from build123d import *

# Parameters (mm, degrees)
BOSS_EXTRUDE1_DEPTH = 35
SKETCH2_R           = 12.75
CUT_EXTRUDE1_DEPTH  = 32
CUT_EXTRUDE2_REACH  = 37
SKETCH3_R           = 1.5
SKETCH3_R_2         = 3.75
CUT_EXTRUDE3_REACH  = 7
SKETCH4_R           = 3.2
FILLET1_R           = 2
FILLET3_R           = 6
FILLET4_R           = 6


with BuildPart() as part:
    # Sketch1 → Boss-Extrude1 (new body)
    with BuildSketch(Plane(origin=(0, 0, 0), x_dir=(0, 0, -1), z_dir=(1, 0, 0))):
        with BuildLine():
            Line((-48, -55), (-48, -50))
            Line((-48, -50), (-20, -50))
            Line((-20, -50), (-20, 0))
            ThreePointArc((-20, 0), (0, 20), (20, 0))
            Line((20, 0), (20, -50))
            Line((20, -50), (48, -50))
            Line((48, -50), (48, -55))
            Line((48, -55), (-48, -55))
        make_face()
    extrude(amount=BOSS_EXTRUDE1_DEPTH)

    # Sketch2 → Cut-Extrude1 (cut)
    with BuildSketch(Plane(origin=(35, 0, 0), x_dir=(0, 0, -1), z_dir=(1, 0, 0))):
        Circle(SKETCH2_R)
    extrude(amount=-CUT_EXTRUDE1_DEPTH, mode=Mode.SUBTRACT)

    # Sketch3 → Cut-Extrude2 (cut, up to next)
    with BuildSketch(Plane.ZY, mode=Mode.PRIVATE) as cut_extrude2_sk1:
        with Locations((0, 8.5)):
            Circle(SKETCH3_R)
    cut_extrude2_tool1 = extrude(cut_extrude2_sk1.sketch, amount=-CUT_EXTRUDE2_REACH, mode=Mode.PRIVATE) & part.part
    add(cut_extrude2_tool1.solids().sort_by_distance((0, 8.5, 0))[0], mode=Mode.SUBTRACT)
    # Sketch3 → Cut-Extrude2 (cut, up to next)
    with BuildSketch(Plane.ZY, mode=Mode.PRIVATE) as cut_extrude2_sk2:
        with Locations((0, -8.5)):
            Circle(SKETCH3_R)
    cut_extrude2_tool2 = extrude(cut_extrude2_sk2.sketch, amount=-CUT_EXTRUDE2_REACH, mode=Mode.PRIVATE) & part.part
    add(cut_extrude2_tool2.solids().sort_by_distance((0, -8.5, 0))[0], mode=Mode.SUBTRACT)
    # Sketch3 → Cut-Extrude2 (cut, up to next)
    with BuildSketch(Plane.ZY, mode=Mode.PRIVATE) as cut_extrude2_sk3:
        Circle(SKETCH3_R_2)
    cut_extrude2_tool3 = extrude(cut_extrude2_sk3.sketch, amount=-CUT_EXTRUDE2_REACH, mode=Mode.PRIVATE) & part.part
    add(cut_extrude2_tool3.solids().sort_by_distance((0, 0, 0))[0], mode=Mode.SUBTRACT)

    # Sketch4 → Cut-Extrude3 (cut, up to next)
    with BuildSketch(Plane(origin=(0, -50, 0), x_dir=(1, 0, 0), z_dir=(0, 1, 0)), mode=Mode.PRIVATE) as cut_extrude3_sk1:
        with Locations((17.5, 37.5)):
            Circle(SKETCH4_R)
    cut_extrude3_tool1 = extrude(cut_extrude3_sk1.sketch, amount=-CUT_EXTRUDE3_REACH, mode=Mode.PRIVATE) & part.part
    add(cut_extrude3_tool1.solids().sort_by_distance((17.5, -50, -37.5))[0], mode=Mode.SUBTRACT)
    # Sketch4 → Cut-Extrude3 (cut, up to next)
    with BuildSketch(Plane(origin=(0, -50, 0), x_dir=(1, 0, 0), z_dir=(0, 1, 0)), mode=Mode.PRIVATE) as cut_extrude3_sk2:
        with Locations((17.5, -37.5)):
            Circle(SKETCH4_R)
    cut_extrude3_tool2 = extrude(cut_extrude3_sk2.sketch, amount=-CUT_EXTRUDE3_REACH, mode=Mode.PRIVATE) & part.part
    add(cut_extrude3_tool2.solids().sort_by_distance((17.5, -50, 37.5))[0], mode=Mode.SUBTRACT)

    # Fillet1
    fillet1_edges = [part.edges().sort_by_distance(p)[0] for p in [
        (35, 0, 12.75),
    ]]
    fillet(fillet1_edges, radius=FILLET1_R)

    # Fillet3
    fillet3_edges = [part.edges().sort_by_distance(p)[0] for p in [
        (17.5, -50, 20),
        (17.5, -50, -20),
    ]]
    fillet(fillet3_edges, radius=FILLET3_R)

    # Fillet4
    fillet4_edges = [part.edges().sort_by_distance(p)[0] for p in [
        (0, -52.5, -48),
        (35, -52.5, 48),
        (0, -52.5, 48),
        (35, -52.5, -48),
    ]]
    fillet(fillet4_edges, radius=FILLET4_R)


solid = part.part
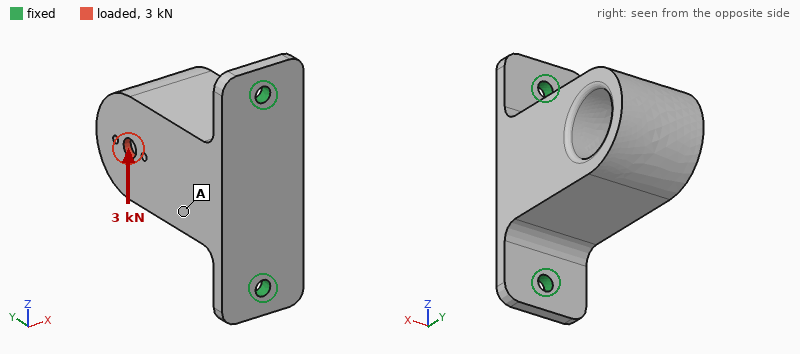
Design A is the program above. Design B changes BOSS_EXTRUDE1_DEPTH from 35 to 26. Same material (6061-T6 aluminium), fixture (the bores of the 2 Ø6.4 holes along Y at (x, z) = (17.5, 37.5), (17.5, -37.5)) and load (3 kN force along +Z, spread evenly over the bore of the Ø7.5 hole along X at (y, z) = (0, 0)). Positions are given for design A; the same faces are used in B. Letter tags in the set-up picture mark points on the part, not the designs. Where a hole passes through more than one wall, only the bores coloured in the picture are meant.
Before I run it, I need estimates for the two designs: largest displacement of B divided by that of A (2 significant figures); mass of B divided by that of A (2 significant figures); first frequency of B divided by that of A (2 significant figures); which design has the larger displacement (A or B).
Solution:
1.2
0.75
0.97
B
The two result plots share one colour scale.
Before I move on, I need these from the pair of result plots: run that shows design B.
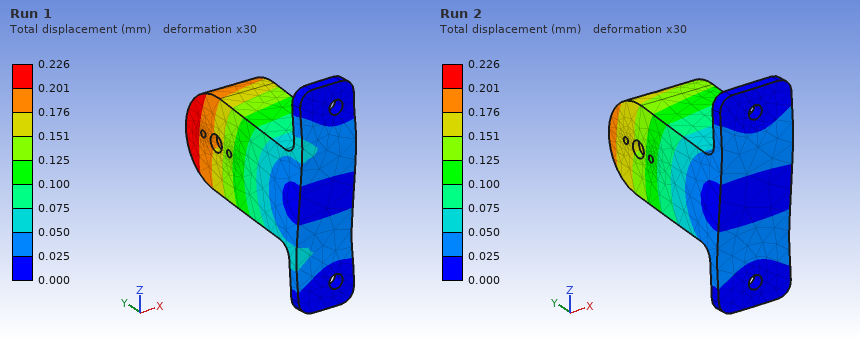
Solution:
Run 1
